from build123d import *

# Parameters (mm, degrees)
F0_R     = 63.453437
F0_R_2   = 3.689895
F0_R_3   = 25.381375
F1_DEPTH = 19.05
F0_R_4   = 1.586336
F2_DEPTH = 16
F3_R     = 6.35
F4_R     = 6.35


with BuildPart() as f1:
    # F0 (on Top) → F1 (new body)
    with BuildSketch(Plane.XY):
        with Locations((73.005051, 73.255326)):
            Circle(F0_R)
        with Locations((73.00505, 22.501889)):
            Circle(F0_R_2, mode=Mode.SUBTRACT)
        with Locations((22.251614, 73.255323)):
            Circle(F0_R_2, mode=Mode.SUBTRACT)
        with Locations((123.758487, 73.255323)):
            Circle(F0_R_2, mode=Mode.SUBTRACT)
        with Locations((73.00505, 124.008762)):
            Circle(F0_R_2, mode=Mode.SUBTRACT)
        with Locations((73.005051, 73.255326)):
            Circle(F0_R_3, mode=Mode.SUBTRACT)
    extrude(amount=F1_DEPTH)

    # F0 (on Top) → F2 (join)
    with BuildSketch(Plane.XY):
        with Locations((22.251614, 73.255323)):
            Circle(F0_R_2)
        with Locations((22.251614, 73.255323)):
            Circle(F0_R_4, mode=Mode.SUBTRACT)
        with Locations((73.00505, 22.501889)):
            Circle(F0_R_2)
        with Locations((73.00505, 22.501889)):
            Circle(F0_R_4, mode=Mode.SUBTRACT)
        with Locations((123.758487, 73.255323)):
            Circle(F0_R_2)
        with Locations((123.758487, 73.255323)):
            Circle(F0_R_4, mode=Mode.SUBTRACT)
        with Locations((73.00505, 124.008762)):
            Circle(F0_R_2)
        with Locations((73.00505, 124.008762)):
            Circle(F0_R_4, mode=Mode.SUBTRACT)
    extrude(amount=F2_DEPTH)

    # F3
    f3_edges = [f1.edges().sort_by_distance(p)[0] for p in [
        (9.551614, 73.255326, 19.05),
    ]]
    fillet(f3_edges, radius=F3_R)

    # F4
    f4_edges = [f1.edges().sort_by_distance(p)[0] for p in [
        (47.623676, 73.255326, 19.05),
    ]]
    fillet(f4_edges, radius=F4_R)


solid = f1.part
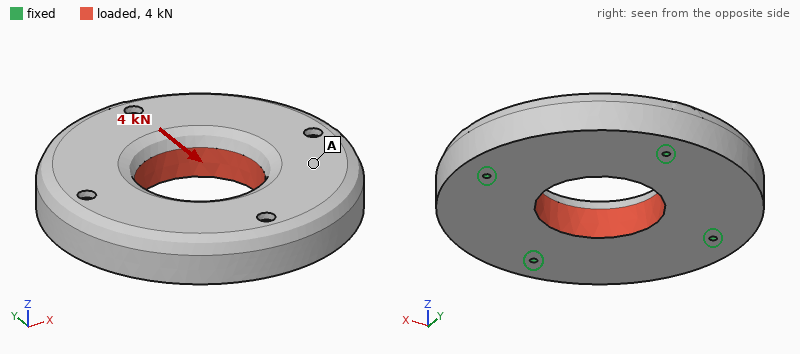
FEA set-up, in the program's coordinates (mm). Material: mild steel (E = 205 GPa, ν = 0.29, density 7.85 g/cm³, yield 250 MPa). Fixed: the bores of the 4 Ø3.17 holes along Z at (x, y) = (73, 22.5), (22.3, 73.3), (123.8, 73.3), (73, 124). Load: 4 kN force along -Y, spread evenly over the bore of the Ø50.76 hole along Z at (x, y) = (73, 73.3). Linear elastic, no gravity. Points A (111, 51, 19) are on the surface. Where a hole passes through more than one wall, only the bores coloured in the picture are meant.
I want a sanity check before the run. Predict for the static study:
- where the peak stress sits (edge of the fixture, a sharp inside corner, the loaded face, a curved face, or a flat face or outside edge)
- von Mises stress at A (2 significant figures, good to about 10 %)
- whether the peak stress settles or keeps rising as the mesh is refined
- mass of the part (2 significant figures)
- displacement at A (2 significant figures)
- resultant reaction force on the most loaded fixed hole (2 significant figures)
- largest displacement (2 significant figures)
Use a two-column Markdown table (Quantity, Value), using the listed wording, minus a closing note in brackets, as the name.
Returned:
| Quantity | Value |
|---|---|
| where the peak stress sits | edge of the fixture |
| von Mises stress at A | 0.83 MPa |
| whether the peak stress settles or keeps rising as the mesh is refined | keeps rising |
| mass of the part | 1.5 kg |
| displacement at A | 0.29 µm |
| resultant reaction force on the most loaded fixed hole | 1.1 kN |
| largest displacement | 0.56 µm |
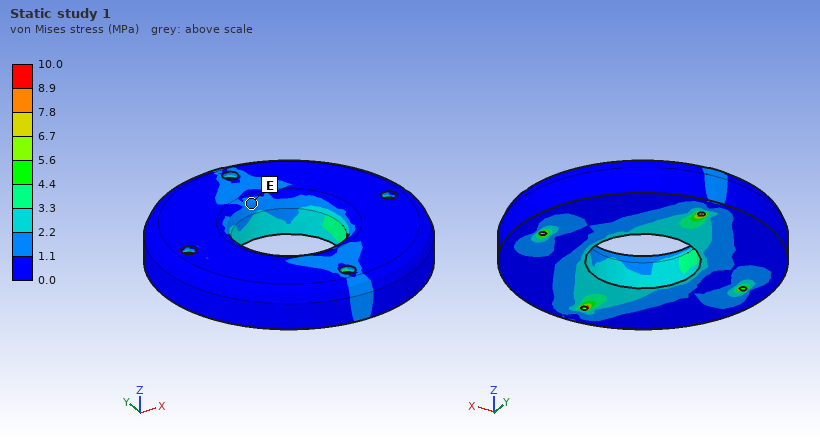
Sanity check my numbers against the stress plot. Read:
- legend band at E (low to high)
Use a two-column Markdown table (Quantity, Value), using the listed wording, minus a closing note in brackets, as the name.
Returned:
| Quantity | Value |
|---|---|
| legend band at E | 1.1 to 2.2 MPa |
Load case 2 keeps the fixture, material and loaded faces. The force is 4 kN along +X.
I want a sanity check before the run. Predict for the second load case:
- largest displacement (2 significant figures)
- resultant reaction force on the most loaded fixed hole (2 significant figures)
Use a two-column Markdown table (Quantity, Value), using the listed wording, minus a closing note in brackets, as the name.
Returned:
| Quantity | Value |
|---|---|
| largest displacement | 0.56 µm |
| resultant reaction force on the most loaded fixed hole | 1.1 kN |
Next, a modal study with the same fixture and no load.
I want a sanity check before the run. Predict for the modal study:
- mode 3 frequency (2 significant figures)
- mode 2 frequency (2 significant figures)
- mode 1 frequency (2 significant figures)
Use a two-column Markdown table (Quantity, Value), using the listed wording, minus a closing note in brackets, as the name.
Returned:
| Quantity | Value |
|---|---|
| mode 3 frequency | 9000 Hz |
| mode 2 frequency | 9000 Hz |
| mode 1 frequency | 7400 Hz |
